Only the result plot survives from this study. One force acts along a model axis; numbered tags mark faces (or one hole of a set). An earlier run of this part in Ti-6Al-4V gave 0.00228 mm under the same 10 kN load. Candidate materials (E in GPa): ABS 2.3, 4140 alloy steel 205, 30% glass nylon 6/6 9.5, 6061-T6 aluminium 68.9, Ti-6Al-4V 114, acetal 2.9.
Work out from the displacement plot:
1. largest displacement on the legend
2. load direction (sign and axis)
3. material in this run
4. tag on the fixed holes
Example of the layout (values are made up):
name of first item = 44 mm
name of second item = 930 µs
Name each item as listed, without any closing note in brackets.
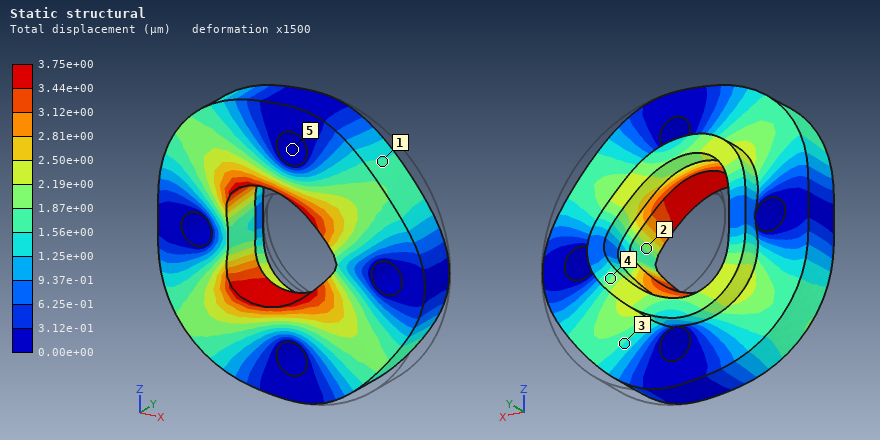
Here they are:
largest displacement on the legend = 3.75e+00 µm
load direction = -X
material in this run = 6061-T6 aluminium
tag on the fixed holes = 5
